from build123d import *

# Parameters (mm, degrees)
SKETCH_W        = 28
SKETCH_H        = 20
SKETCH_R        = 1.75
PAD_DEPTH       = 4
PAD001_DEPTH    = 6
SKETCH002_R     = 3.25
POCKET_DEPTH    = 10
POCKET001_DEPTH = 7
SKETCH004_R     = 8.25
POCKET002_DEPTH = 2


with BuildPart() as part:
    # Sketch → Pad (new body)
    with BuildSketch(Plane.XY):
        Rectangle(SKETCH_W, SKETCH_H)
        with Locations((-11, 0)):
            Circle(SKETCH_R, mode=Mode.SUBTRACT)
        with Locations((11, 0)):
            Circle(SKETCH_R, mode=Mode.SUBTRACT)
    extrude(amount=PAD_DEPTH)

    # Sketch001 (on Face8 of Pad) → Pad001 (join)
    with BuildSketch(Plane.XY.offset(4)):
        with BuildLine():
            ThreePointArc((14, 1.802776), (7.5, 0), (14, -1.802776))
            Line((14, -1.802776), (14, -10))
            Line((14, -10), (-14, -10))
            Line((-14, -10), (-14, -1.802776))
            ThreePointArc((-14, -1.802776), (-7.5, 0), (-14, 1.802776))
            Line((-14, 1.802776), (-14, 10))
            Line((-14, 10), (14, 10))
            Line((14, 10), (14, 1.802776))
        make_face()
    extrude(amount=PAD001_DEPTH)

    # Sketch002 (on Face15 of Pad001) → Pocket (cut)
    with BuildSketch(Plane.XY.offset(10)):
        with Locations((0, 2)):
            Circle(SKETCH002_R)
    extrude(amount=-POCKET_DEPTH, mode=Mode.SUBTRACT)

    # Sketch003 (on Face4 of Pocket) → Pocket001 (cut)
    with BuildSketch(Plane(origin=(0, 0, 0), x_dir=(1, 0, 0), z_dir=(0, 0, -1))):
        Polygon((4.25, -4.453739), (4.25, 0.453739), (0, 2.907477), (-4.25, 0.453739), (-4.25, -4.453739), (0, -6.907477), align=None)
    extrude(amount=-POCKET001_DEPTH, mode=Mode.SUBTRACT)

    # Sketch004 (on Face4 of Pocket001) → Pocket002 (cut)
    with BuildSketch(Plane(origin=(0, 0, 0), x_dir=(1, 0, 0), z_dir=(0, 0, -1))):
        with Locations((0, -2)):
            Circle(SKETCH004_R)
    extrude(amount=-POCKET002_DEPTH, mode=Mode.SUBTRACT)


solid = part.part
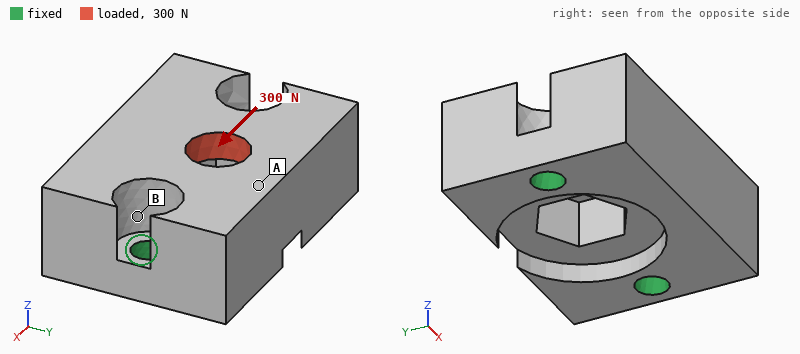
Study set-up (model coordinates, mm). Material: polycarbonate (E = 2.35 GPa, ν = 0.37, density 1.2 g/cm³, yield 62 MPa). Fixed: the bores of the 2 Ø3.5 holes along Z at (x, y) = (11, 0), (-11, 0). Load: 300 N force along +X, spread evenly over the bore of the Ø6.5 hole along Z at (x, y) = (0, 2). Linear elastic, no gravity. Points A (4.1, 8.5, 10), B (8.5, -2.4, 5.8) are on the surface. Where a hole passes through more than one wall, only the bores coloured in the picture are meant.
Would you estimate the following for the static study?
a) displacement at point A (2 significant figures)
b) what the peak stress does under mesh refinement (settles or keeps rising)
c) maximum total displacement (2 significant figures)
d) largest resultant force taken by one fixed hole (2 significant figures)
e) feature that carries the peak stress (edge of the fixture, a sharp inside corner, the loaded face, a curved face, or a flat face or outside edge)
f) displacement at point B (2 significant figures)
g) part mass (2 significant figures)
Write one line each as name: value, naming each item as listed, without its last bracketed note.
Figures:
displacement at point A: 29 µm
what the peak stress does under mesh refinement: keeps rising
maximum total displacement: 42 µm
largest resultant force taken by one fixed hole: 170 N
feature that carries the peak stress: edge of the fixture
displacement at point B: 16 µm
part mass: 5.1 g
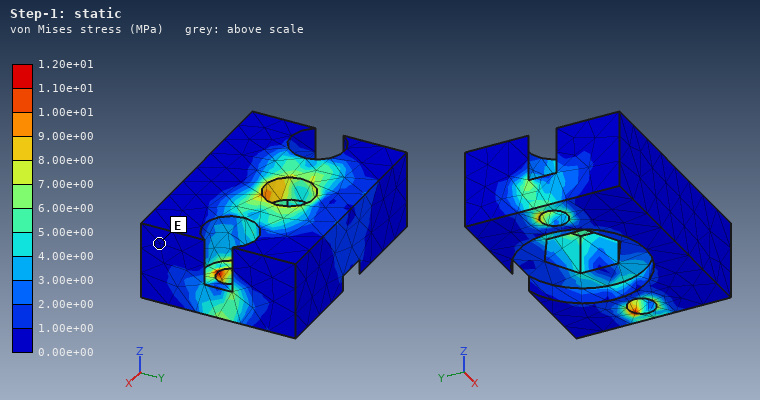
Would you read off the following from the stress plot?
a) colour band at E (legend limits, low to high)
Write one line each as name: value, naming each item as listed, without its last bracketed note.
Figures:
colour band at E: 0.00e+00 to 1.00e+00 MPa
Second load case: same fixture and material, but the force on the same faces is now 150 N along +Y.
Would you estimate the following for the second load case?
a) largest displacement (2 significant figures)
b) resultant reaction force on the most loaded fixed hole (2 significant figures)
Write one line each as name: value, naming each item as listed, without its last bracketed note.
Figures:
largest displacement: 95 µm
resultant reaction force on the most loaded fixed hole: 75 N
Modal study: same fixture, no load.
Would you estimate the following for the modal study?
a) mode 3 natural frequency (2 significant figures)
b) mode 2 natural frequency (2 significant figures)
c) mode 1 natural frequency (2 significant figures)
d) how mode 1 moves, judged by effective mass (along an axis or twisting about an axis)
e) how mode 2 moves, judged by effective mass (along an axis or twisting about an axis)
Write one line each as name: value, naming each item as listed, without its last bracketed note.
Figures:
mode 3 natural frequency: 8700 Hz
mode 2 natural frequency: 8100 Hz
mode 1 natural frequency: 3900 Hz
how mode 1 moves, judged by effective mass: along Y
how mode 2 moves, judged by effective mass: along Z
